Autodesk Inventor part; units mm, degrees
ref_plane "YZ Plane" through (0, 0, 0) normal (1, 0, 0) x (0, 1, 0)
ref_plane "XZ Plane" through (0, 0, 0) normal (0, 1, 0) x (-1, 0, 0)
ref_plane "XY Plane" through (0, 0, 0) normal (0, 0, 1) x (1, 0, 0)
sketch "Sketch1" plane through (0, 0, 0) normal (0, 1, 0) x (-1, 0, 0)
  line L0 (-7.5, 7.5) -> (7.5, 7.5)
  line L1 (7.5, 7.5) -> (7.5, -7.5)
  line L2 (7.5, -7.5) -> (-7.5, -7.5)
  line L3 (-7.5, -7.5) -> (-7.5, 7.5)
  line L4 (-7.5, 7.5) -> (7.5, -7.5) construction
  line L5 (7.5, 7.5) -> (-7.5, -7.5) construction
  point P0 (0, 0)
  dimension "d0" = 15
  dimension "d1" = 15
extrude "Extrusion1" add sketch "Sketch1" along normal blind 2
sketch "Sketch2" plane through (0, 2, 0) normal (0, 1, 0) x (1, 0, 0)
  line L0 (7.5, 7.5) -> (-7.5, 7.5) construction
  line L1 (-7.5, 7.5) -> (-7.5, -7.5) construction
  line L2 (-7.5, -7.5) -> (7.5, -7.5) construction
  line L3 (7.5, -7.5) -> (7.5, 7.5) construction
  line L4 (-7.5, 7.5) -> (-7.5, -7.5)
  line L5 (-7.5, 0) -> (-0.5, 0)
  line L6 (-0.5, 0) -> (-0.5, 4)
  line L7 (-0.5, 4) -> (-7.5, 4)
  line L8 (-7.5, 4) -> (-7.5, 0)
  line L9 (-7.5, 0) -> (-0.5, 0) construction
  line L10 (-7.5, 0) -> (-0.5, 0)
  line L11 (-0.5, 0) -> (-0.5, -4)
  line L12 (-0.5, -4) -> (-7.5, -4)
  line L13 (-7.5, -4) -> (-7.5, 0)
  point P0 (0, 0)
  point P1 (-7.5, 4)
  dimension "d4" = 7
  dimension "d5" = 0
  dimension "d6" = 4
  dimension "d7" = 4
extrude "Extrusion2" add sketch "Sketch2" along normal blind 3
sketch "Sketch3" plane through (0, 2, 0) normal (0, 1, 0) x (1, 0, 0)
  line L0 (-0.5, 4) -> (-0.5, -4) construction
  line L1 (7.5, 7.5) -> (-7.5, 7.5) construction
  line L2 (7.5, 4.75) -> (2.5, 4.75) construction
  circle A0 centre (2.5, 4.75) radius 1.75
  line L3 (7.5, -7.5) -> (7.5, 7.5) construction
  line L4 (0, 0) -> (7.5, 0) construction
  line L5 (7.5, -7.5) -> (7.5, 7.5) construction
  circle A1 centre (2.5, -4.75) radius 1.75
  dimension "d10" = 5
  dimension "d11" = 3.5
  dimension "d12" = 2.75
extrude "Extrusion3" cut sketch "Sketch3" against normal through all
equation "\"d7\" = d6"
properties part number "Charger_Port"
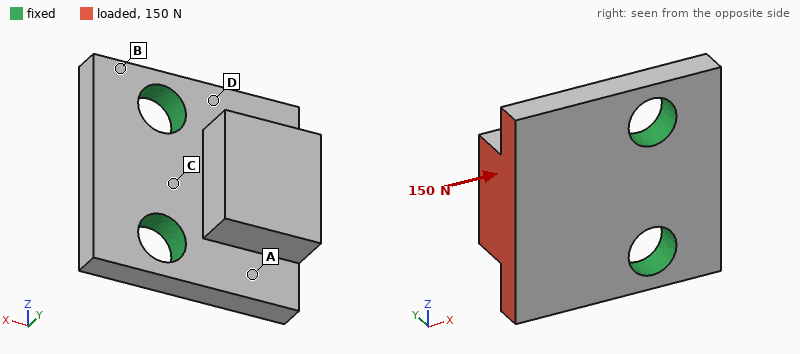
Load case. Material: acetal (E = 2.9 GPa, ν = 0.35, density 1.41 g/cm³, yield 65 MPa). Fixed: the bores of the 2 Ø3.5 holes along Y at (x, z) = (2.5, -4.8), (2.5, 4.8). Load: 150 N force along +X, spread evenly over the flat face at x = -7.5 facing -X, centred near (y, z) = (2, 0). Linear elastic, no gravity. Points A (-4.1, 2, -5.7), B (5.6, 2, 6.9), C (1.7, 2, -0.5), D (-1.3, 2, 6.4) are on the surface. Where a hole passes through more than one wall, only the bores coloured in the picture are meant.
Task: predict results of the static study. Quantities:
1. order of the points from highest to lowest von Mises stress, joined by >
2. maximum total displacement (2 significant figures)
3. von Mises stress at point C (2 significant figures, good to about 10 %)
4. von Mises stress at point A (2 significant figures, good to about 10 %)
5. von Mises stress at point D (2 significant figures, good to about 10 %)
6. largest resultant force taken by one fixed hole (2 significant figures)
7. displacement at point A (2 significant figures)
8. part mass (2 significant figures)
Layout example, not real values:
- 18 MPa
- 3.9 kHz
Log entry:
- D > C > A > B
- 0.15 mm
- 9.7 MPa
- 5.9 MPa
- 13 MPa
- 77 N
- 0.066 mm
- 0.82 g
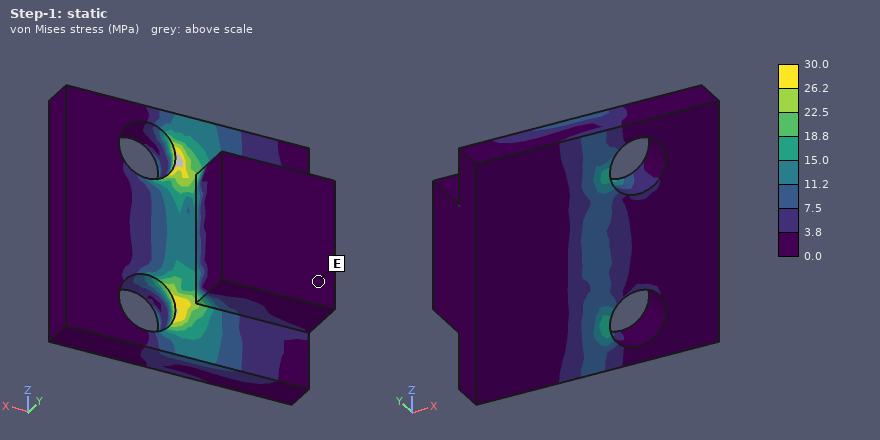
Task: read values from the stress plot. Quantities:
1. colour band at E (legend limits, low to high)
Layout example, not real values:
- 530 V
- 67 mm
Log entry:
- 0.0 to 3.8 MPa
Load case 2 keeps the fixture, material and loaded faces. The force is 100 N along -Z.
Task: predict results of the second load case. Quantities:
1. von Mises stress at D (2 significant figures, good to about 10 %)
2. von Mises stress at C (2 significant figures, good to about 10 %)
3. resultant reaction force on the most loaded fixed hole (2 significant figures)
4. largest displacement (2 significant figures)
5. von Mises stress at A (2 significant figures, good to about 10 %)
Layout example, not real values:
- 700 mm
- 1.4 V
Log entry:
- 7.0 MPa
- 2.5 MPa
- 99 N
- 47 µm
- 4.9 MPa
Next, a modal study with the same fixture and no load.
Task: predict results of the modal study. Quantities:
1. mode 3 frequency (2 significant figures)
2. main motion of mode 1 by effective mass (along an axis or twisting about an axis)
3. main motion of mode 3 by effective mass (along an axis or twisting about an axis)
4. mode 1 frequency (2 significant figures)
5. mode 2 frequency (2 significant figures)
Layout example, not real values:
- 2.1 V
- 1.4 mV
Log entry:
- 16 kHz
- along Y
- along Z
- 4300 Hz
- 12 kHz
